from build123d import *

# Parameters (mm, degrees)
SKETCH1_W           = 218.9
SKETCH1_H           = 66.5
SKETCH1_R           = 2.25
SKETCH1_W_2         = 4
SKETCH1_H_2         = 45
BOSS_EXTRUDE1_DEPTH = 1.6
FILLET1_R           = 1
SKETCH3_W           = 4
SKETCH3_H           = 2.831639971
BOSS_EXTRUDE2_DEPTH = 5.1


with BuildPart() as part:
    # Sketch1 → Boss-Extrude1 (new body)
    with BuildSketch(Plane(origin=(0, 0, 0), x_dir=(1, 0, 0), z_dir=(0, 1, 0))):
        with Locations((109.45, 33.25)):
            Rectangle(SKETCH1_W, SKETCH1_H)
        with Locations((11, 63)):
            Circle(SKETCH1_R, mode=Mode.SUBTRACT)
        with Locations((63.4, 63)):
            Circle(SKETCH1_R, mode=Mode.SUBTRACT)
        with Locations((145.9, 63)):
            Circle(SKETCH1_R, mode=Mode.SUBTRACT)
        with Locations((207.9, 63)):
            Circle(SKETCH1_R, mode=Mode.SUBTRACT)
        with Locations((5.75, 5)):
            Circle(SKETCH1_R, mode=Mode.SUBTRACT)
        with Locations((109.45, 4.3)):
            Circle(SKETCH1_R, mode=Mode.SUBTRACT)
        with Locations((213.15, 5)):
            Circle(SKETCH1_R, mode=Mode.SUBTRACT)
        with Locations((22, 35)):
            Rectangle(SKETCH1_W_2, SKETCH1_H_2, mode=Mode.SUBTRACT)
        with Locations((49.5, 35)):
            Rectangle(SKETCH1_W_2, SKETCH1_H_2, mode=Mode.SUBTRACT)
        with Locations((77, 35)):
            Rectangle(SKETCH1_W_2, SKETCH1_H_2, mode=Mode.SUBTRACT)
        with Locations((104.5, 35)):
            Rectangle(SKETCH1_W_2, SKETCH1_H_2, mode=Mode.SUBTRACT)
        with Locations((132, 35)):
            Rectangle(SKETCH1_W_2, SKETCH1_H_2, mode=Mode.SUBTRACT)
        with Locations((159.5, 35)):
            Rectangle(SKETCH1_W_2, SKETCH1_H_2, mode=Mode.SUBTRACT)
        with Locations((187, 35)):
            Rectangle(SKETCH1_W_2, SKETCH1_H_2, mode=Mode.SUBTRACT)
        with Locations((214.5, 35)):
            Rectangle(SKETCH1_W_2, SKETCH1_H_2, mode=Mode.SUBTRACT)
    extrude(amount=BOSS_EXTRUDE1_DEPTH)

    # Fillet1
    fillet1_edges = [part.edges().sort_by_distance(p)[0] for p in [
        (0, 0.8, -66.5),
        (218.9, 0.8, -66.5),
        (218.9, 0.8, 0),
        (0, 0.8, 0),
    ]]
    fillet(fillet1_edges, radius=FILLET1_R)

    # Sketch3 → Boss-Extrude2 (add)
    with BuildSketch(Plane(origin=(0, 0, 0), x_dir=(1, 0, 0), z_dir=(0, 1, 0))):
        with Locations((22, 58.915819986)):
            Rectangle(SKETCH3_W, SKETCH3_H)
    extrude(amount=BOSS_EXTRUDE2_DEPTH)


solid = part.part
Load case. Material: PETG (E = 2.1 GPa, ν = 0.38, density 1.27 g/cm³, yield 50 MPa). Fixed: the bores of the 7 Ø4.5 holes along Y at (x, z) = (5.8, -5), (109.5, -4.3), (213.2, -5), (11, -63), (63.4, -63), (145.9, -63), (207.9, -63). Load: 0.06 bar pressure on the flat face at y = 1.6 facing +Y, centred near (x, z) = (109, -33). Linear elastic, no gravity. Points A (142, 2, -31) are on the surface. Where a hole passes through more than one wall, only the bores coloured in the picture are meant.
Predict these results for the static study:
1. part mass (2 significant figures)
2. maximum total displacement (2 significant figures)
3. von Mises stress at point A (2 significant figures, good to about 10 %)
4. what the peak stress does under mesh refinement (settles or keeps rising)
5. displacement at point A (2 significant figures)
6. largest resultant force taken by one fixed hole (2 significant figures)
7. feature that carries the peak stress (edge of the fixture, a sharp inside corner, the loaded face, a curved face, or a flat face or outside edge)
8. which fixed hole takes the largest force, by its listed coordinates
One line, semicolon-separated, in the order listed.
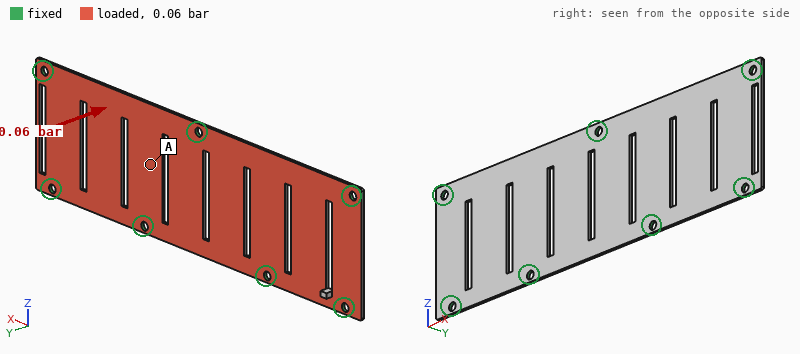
26 g; 2.5 mm; 2.9 MPa; keeps rising; 1.1 mm; 18 N; edge of the fixture; (109.5, -4.3)
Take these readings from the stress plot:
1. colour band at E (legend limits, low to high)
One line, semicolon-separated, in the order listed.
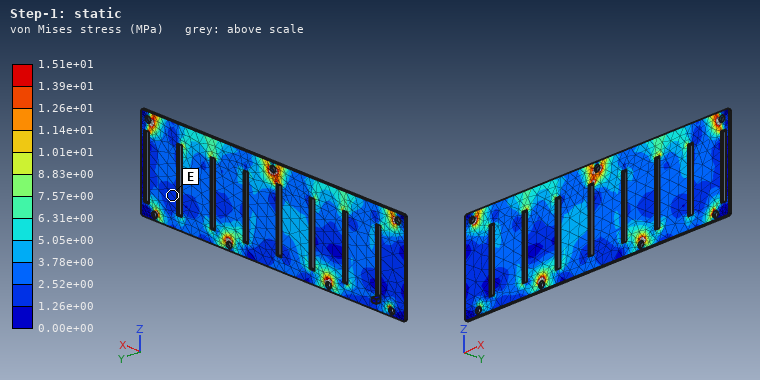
1.26e+00 to 2.52e+00 MPa
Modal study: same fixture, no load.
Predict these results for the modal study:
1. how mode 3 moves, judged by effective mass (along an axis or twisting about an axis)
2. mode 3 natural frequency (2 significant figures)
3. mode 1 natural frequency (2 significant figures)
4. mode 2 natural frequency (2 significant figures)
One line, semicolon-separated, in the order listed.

along Y; 300 Hz; 210 Hz; 220 Hz
